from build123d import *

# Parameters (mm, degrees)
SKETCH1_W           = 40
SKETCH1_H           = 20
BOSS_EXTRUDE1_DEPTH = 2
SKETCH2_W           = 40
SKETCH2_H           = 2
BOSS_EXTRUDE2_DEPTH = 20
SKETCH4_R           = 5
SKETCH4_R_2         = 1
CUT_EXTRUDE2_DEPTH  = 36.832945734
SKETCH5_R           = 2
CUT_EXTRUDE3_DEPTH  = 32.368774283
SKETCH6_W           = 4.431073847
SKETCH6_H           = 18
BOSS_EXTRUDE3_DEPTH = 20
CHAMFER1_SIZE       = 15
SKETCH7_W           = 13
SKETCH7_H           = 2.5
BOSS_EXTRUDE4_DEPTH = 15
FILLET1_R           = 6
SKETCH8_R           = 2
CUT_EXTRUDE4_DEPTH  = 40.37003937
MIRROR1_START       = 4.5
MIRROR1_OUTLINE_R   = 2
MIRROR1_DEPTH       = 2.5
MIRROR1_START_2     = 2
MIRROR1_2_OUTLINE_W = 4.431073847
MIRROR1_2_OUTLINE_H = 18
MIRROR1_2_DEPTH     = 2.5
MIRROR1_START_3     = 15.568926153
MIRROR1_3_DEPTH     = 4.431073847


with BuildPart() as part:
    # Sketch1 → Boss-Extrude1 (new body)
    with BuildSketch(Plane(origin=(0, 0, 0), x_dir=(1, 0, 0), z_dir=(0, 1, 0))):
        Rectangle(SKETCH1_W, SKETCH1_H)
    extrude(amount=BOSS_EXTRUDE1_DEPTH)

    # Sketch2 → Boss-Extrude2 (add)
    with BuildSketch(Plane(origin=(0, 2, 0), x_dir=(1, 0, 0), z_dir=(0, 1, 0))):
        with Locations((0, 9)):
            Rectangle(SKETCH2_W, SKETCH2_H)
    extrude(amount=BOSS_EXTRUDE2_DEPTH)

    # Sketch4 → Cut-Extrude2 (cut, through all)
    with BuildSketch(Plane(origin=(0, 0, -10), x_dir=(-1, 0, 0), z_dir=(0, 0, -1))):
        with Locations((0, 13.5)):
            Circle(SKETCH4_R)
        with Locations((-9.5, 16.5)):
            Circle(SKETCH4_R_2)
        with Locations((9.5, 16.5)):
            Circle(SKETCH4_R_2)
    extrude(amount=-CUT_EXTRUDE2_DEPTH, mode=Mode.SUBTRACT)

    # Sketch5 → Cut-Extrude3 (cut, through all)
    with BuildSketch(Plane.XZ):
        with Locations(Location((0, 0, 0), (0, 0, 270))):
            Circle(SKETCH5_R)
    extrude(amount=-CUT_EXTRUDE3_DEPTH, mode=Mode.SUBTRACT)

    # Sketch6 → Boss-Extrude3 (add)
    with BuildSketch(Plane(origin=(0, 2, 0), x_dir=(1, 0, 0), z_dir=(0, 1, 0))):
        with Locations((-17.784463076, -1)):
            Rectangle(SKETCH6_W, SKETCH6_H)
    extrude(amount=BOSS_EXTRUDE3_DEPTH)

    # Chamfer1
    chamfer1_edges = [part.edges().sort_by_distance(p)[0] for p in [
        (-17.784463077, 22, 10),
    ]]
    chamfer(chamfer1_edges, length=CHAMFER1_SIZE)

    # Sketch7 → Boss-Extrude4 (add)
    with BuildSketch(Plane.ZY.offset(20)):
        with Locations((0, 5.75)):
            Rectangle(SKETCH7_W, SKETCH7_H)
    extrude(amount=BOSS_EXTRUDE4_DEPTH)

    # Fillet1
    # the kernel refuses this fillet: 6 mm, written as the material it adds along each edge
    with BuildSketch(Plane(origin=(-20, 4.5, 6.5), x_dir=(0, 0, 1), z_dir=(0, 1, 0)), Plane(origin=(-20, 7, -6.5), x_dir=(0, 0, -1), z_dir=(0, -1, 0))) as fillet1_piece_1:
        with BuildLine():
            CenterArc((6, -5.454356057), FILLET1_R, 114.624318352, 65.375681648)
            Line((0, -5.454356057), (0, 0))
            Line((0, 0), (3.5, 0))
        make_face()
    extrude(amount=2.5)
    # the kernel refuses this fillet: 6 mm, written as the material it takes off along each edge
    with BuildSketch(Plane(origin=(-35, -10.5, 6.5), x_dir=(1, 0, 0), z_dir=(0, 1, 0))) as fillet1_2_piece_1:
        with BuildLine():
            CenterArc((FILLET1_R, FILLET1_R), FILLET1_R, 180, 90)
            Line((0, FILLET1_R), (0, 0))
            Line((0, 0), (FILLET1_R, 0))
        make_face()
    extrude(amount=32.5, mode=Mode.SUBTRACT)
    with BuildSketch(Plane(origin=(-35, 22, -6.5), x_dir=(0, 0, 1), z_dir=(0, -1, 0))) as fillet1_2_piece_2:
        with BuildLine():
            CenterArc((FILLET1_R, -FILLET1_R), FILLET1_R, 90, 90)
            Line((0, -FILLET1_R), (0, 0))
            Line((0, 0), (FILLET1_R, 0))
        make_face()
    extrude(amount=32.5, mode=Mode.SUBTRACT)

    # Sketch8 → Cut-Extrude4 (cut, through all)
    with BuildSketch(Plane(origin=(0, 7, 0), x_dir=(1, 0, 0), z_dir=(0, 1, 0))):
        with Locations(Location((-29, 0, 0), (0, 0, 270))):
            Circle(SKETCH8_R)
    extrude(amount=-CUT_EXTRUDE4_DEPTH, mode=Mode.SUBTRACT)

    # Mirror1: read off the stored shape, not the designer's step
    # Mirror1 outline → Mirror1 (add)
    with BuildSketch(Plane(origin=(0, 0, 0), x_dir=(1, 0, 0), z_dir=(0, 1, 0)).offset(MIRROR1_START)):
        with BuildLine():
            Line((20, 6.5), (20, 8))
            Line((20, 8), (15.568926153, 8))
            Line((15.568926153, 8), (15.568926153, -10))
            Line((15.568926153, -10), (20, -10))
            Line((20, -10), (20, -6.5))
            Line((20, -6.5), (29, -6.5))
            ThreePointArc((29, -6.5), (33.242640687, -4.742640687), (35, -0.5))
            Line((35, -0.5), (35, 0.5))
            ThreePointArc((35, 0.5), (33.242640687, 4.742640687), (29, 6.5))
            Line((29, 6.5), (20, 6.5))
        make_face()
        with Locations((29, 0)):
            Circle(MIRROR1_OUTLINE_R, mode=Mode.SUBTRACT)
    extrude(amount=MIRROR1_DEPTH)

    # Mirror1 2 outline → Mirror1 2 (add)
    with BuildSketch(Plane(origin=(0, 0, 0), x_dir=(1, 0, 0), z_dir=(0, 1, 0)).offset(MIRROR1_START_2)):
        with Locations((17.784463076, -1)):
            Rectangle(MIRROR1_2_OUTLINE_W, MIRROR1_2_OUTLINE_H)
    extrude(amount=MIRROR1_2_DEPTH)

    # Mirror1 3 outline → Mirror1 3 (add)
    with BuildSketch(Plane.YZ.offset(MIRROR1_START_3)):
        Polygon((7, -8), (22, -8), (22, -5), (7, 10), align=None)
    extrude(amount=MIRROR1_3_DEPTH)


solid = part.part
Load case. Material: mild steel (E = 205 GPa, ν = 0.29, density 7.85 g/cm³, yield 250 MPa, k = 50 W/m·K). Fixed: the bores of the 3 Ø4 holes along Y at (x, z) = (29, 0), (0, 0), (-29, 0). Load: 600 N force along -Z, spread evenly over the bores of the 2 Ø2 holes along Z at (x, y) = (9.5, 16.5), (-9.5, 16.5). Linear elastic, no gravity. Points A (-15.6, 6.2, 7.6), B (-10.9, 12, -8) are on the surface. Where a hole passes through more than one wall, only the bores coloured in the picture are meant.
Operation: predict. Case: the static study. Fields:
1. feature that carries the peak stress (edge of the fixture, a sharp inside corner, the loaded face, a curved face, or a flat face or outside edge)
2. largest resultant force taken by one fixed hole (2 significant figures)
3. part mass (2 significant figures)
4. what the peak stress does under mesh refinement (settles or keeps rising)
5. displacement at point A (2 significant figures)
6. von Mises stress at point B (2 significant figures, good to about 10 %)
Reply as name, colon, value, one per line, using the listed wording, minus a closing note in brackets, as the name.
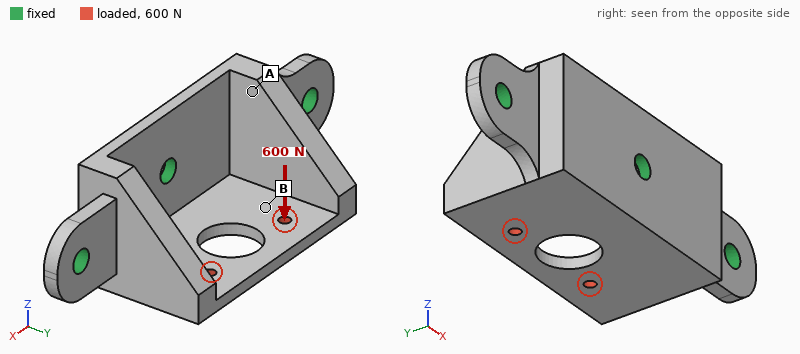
feature that carries the peak stress: edge of the fixture
largest resultant force taken by one fixed hole: 630 N
part mass: 48 g
what the peak stress does under mesh refinement: keeps rising
displacement at point A: 13 µm
von Mises stress at point B: 60 MPa
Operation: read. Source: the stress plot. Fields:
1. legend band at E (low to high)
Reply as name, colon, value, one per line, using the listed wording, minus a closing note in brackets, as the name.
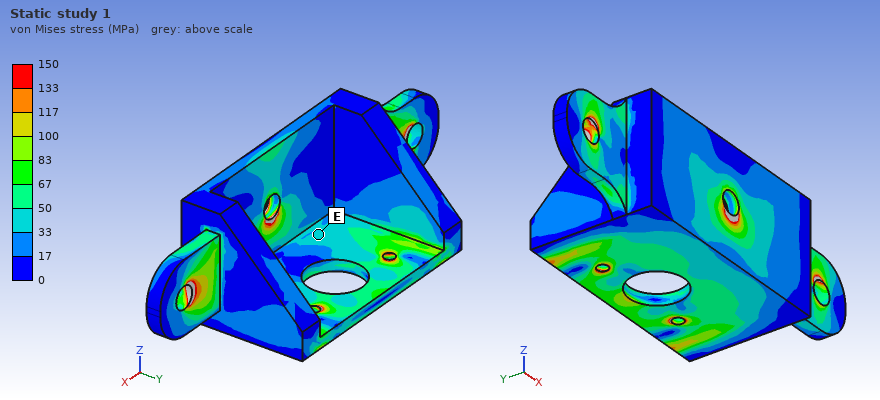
legend band at E: 33 to 50 MPa
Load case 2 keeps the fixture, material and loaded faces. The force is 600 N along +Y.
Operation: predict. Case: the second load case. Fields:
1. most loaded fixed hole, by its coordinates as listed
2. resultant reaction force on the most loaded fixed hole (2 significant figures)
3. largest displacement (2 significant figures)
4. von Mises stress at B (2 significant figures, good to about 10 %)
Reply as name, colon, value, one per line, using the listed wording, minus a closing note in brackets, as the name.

most loaded fixed hole, by its coordinates as listed: (0, 0)
resultant reaction force on the most loaded fixed hole: 480 N
largest displacement: 27 µm
von Mises stress at B: 16 MPa
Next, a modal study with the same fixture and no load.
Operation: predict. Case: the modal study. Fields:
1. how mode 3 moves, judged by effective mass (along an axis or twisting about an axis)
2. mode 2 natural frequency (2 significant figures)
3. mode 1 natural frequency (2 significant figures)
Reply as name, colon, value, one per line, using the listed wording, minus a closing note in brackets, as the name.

how mode 3 moves, judged by effective mass: along Y
mode 2 natural frequency: 6300 Hz
mode 1 natural frequency: 5300 Hz
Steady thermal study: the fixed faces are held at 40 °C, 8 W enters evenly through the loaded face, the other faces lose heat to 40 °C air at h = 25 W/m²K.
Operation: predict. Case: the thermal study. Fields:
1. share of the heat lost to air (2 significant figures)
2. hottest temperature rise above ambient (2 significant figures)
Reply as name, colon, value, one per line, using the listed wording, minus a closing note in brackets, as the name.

share of the heat lost to air: 19 %
hottest temperature rise above ambient: 40 K
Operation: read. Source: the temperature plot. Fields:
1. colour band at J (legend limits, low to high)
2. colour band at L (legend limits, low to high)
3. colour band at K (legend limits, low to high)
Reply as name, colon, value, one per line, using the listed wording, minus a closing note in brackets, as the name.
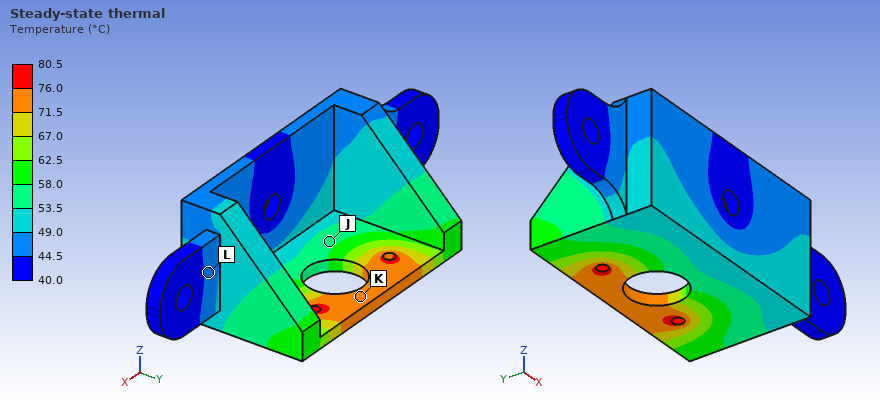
colour band at J: 53.5 to 58.0 °C
colour band at L: 44.5 to 49.0 °C
colour band at K: 71.5 to 76.0 °C
